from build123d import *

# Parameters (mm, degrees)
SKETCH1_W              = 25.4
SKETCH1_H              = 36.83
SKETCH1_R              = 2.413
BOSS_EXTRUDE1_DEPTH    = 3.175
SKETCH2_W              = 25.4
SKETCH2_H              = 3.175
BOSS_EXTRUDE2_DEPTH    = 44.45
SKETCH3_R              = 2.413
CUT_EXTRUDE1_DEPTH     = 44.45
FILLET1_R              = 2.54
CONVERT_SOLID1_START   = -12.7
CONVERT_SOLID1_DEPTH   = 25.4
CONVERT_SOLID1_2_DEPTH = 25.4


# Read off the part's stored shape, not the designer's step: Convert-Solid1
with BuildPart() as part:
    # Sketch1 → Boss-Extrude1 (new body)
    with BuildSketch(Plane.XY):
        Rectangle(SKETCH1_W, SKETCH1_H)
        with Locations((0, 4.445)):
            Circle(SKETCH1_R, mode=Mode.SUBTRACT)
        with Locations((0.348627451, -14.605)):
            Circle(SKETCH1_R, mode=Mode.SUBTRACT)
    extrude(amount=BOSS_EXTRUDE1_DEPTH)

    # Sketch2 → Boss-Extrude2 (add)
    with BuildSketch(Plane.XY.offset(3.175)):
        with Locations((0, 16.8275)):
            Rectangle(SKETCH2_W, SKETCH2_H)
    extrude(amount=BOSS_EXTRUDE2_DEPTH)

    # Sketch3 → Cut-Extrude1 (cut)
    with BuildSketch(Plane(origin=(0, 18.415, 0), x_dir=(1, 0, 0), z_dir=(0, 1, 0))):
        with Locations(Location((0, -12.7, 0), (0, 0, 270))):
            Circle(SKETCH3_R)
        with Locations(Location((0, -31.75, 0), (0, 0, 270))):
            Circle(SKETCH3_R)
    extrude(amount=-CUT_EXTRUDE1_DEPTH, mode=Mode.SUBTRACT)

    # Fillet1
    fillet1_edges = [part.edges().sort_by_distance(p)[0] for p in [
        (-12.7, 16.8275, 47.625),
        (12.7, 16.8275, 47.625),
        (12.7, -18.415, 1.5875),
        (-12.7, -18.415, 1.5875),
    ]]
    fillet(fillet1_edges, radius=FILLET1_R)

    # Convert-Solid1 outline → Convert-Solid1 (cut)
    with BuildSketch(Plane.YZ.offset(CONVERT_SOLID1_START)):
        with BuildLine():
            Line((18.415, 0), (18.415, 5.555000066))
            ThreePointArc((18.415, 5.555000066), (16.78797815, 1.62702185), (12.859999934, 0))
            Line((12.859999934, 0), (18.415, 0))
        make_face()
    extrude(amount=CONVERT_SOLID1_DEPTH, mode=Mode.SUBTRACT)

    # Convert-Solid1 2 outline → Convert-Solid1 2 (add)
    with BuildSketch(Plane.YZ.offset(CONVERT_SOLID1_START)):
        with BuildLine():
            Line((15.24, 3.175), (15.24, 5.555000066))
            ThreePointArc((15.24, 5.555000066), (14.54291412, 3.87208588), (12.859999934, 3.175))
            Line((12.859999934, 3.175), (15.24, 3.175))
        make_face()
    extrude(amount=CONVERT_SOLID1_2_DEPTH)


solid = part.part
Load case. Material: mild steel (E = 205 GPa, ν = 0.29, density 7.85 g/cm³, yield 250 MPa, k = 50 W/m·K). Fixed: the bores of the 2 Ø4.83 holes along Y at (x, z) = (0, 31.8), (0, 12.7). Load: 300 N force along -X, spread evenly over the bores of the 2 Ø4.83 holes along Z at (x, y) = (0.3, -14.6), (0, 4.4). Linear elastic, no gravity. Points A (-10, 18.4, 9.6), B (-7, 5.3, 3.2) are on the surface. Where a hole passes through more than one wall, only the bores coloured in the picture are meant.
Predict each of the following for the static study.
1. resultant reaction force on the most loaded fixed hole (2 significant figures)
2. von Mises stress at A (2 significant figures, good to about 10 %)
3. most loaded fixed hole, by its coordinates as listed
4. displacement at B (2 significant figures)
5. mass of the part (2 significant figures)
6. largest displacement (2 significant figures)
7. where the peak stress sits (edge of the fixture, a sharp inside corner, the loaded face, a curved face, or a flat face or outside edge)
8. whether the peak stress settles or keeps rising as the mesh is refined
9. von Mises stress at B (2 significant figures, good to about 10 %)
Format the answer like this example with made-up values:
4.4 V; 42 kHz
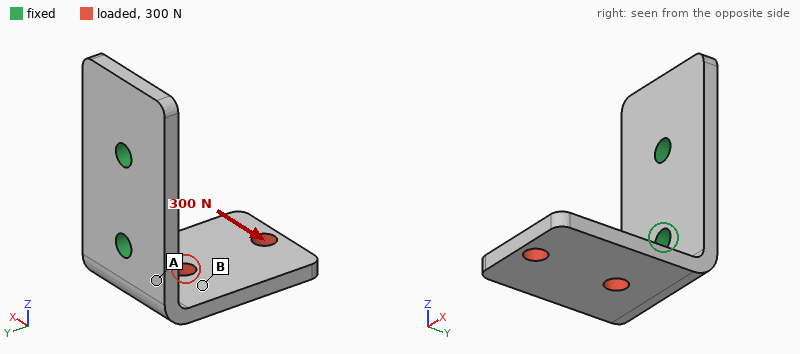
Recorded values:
410 N; 56 MPa; (0, 12.7); 37 µm; 48 g; 100 µm; edge of the fixture; keeps rising; 26 MPa
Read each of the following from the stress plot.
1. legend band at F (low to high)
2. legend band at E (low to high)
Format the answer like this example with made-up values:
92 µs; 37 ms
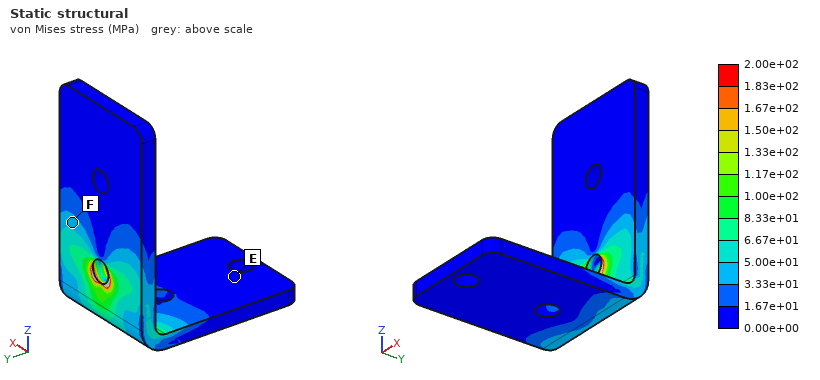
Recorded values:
3.33e+01 to 5.00e+01 MPa; 0.00e+00 to 1.67e+01 MPa
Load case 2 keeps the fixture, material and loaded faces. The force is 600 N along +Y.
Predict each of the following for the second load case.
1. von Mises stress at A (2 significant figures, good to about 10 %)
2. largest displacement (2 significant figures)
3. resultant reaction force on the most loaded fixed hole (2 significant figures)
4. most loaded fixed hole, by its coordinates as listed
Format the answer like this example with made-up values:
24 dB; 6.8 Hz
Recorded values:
60 MPa; 93 µm; 670 N; (0, 12.7)
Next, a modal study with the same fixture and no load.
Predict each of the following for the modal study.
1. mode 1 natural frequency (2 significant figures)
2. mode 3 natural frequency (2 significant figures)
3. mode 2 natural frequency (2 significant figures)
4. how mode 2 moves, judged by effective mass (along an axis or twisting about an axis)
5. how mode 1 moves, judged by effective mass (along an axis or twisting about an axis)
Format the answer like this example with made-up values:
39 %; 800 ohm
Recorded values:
1500 Hz; 6000 Hz; 2500 Hz; along X; along Z
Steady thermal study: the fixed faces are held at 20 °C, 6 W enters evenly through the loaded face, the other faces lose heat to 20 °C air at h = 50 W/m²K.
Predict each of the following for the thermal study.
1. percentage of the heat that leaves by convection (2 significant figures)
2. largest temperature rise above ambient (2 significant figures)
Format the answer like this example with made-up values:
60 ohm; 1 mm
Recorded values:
42 %; 36 K
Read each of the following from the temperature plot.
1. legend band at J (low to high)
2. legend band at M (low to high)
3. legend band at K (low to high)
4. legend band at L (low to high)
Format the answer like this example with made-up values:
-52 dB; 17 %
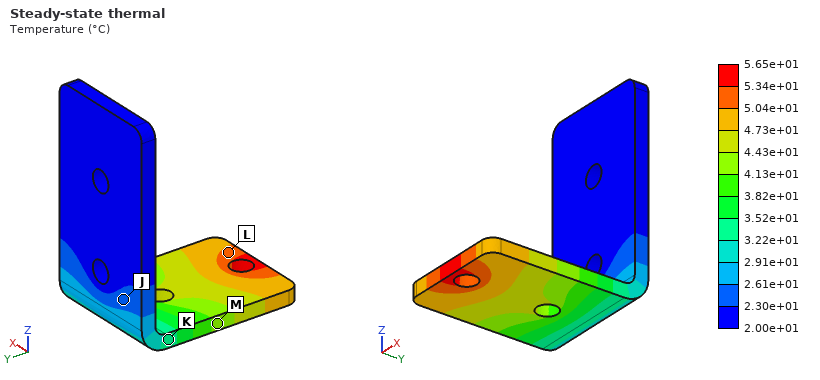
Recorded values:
2.30e+01 to 2.61e+01 °C; 4.13e+01 to 4.43e+01 °C; 3.22e+01 to 3.52e+01 °C; 5.04e+01 to 5.34e+01 °C
